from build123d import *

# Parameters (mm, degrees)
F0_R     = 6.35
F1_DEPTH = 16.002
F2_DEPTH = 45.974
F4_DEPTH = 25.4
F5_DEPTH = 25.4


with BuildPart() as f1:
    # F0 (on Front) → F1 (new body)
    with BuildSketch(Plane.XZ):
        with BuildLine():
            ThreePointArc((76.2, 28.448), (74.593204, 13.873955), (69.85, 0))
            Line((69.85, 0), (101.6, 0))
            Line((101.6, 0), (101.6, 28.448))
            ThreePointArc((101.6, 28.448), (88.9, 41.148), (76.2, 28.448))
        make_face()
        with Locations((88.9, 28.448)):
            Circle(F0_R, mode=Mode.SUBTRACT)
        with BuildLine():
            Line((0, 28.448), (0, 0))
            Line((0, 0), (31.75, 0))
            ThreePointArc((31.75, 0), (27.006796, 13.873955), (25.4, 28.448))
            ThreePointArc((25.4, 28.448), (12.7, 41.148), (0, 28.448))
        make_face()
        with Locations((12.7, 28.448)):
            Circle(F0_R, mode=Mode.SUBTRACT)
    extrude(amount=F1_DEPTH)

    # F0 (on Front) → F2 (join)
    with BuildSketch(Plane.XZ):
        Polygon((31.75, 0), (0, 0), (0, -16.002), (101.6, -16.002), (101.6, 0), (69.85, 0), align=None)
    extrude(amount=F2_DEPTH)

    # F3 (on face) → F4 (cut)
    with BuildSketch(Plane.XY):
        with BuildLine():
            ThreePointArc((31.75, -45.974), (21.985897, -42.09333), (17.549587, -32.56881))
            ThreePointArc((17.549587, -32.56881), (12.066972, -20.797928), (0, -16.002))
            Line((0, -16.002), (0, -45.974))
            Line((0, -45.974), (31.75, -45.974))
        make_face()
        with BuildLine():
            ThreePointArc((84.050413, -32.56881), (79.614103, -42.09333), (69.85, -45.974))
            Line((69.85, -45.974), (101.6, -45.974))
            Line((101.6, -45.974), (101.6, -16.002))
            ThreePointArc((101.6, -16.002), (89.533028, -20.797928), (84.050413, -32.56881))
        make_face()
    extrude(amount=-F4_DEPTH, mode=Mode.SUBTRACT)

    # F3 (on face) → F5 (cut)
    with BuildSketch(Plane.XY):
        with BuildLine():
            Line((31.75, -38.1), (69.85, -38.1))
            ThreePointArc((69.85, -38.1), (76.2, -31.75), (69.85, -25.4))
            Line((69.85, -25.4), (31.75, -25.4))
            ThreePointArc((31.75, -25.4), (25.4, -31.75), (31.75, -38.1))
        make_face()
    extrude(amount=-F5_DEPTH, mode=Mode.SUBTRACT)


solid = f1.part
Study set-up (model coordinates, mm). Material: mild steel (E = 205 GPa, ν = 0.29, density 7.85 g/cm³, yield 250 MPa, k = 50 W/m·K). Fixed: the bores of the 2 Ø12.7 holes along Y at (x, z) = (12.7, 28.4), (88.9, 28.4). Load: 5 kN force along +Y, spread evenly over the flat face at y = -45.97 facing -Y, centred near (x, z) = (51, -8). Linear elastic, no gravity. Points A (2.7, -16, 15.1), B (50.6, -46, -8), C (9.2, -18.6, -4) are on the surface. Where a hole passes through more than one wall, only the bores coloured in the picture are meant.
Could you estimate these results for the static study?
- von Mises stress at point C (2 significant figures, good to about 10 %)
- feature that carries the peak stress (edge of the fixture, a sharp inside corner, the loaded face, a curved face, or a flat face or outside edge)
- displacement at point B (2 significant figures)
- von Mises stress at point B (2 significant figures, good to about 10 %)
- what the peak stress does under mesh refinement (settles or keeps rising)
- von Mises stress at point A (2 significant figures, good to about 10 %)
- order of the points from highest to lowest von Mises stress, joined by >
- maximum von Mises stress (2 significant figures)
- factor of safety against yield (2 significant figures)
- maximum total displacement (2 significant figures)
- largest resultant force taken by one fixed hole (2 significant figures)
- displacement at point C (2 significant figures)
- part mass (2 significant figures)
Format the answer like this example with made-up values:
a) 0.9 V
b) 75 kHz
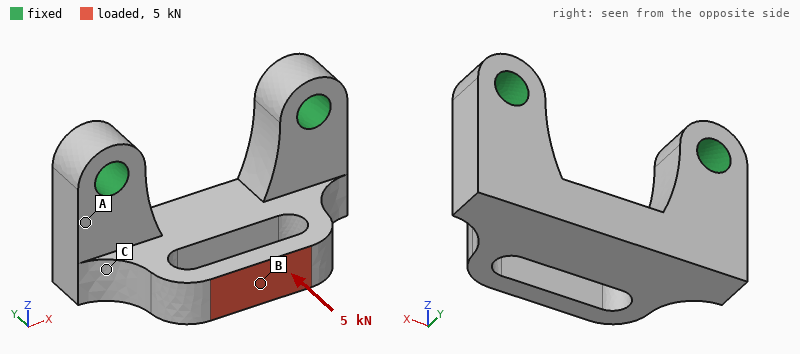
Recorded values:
a) 16 MPa
b) a curved face
c) 60 µm
d) 120 MPa
e) settles
f) 44 MPa
g) B > A > C
h) 170 MPa
i) 1.5
j) 67 µm
k) 2.5 kN
l) 17 µm
m) 610 g
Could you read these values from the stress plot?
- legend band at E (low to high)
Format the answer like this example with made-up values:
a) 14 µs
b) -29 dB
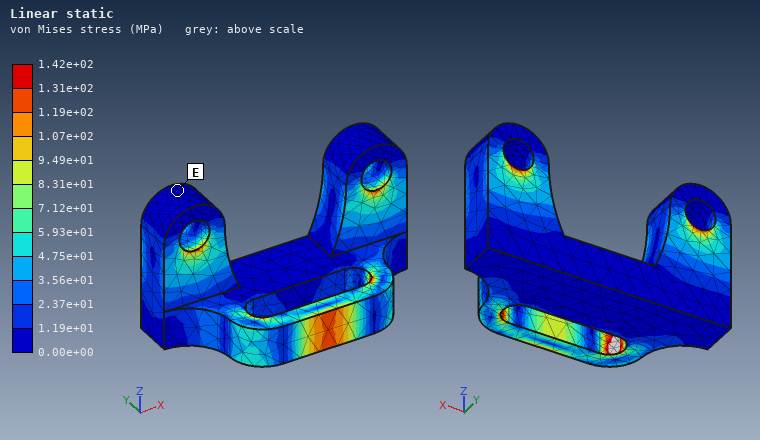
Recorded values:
a) 0.00e+00 to 1.19e+01 MPa
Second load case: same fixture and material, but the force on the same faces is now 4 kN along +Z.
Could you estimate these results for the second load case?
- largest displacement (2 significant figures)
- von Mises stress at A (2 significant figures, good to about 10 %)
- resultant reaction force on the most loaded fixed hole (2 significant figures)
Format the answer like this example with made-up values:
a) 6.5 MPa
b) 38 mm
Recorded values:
a) 0.11 mm
b) 57 MPa
c) 2.2 kN
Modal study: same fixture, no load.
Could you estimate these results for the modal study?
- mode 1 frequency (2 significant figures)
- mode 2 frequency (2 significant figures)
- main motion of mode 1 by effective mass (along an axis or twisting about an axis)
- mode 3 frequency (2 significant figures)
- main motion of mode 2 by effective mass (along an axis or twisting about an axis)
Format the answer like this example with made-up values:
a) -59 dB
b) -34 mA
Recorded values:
a) 3200 Hz
b) 5700 Hz
c) along Y
d) 7200 Hz
e) along X
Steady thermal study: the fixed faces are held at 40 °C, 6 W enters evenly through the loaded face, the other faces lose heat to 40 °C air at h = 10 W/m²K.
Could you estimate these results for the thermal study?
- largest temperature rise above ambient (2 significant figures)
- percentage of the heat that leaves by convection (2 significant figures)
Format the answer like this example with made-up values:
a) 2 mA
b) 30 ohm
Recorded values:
a) 20 K
b) 13 %
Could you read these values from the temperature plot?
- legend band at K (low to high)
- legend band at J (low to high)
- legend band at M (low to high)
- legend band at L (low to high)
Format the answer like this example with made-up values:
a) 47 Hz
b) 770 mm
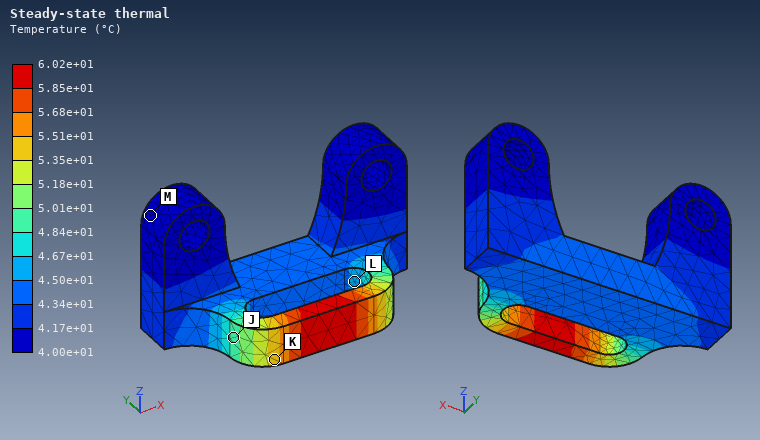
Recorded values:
a) 5.35e+01 to 5.51e+01 °C
b) 4.84e+01 to 5.01e+01 °C
c) 4.00e+01 to 4.17e+01 °C
d) 4.50e+01 to 4.67e+01 °C
